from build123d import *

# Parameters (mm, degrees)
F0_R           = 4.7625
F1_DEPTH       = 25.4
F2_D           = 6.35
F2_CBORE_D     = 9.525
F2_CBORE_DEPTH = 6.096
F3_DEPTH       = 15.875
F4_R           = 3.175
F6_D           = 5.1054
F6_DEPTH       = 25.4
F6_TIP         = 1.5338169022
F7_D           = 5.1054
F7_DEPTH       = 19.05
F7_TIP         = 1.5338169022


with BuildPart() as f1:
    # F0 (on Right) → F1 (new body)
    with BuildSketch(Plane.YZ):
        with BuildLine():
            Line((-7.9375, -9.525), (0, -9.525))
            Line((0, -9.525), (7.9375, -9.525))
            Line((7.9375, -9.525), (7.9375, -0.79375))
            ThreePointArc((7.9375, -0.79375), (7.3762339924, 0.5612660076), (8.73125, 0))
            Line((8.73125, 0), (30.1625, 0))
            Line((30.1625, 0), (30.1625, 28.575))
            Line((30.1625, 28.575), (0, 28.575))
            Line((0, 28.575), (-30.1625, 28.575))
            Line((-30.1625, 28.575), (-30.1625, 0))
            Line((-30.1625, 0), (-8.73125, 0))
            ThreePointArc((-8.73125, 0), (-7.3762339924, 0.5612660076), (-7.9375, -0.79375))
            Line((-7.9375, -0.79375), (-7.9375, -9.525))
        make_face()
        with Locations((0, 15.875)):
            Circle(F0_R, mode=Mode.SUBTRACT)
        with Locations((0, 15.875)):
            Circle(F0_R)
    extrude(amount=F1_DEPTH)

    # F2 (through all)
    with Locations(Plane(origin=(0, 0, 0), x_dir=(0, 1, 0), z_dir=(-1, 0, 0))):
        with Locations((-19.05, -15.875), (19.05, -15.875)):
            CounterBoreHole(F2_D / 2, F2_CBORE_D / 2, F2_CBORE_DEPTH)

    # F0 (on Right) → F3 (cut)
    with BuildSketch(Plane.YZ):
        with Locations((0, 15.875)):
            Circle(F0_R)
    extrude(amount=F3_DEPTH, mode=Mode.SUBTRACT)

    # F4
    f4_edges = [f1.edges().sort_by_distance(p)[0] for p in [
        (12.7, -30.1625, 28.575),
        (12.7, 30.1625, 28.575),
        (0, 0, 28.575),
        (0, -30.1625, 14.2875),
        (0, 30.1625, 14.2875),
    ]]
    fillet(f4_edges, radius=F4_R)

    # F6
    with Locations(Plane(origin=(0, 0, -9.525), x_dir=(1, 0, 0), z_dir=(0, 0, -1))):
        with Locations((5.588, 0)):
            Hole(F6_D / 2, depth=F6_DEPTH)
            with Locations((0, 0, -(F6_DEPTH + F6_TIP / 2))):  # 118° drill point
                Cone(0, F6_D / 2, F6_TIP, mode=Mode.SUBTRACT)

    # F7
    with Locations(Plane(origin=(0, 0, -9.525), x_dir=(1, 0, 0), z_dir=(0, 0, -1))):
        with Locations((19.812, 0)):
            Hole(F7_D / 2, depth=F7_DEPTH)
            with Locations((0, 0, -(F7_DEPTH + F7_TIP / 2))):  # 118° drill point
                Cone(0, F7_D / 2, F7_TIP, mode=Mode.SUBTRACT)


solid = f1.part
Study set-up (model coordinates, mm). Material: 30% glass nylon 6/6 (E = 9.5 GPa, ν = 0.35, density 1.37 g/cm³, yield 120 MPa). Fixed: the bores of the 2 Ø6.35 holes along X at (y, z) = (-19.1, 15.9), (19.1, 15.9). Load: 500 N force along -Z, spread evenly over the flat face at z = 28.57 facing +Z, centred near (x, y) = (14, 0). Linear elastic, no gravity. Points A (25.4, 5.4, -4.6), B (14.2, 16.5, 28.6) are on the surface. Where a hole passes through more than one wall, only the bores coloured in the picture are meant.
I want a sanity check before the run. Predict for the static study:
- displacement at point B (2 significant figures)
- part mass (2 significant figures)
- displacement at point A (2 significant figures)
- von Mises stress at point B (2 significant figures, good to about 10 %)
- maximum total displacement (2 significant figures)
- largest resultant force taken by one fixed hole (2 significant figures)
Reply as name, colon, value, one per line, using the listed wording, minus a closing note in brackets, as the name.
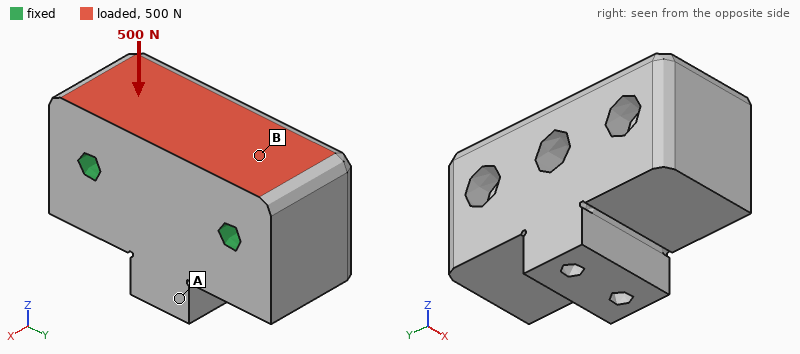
displacement at point B: 0.75 µm
part mass: 59 g
displacement at point A: 0.67 µm
von Mises stress at point B: 0.51 MPa
maximum total displacement: 1.6 µm
largest resultant force taken by one fixed hole: 250 N
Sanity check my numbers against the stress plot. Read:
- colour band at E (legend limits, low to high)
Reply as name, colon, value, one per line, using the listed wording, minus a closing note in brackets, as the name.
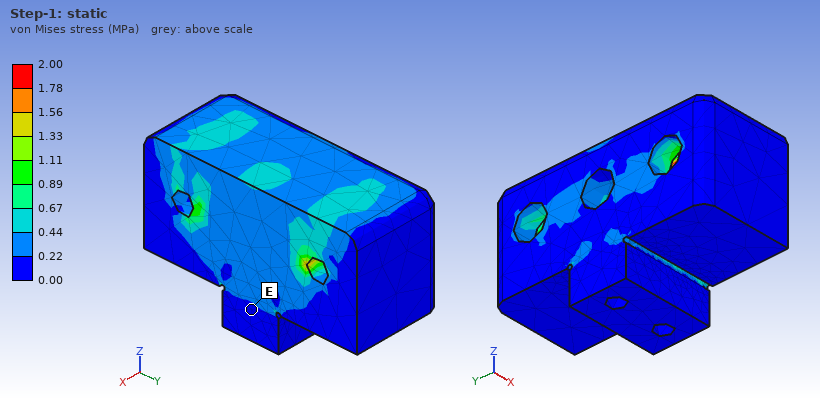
colour band at E: 0.00 to 0.22 MPa
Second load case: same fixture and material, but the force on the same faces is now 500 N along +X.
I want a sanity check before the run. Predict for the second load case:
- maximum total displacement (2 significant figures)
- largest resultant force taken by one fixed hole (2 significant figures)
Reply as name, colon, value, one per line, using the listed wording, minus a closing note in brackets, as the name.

maximum total displacement: 5.7 µm
largest resultant force taken by one fixed hole: 250 N
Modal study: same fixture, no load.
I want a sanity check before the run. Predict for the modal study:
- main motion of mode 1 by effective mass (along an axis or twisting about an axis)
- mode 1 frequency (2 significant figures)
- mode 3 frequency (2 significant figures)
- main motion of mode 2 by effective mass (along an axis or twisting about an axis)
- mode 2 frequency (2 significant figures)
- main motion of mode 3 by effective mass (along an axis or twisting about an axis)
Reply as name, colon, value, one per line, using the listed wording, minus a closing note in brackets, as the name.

main motion of mode 1 by effective mass: along X
mode 1 frequency: 9100 Hz
mode 3 frequency: 15 kHz
main motion of mode 2 by effective mass: along Z
mode 2 frequency: 14 kHz
main motion of mode 3 by effective mass: along Y
